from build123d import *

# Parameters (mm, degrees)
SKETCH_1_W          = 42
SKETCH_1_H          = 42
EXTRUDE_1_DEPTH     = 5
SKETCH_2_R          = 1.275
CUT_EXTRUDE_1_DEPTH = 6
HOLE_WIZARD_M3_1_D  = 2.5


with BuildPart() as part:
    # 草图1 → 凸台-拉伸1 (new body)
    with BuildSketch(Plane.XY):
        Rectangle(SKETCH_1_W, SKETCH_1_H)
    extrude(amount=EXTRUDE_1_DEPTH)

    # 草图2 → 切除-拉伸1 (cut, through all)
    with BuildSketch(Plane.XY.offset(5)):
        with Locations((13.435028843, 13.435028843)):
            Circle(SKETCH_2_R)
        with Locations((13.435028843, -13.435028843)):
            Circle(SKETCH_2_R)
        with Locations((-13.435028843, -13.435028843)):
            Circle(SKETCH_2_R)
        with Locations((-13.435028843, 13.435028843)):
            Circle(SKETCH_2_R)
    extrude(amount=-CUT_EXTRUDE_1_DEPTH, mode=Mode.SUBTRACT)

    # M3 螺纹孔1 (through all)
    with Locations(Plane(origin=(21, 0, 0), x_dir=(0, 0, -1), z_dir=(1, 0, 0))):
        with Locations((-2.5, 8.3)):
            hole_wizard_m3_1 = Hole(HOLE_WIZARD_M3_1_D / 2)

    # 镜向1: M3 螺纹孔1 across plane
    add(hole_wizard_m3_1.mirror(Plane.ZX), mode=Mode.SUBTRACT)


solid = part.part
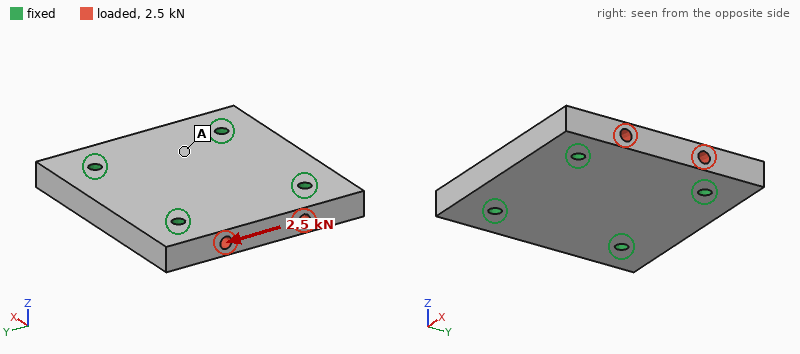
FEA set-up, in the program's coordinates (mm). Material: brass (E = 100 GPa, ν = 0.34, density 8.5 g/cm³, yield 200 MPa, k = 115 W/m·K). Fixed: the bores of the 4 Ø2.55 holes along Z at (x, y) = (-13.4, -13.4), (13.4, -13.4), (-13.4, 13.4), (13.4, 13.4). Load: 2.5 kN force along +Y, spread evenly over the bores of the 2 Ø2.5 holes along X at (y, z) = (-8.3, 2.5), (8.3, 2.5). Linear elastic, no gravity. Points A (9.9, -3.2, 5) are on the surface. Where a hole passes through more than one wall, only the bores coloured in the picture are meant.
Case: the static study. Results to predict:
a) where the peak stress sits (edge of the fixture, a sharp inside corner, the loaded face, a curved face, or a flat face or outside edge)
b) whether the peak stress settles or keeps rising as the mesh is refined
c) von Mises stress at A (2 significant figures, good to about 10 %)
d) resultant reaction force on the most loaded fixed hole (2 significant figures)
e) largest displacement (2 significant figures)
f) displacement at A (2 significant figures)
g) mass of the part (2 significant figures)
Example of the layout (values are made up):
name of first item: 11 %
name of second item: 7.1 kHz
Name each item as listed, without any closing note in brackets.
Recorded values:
where the peak stress sits: edge of the fixture
whether the peak stress settles or keeps rising as the mesh is refined: keeps rising
von Mises stress at A: 3.1 MPa
resultant reaction force on the most loaded fixed hole: 630 N
largest displacement: 1.4 µm
displacement at A: 1.0 µm
mass of the part: 71 g
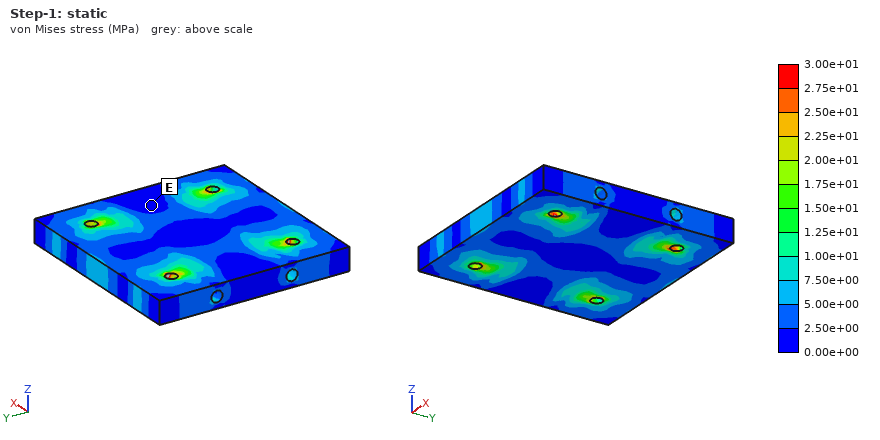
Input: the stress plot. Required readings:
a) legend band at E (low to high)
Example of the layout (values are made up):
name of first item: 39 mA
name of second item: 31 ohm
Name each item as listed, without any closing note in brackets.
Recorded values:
legend band at E: 0.00e+00 to 2.50e+00 MPa
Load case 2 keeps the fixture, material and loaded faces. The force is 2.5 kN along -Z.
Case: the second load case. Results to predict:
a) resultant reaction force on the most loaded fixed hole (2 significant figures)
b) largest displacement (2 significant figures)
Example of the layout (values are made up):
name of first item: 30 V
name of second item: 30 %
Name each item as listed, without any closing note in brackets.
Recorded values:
resultant reaction force on the most loaded fixed hole: 630 N
largest displacement: 8.1 µm
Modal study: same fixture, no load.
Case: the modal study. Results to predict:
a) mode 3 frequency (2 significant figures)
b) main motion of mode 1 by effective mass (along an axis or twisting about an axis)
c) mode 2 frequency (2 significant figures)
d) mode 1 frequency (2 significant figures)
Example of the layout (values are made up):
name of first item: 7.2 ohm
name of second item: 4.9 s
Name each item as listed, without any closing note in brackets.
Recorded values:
mode 3 frequency: 17 kHz
main motion of mode 1 by effective mass: along Z
mode 2 frequency: 17 kHz
mode 1 frequency: 14 kHz
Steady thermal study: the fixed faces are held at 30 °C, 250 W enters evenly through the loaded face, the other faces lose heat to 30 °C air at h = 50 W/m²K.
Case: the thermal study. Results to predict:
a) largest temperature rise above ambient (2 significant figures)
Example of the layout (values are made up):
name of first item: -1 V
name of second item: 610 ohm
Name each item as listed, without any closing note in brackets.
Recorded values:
largest temperature rise above ambient: 60 K
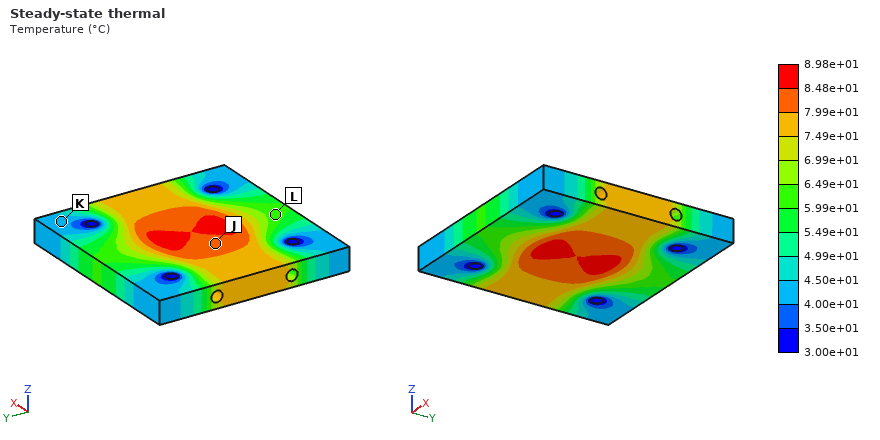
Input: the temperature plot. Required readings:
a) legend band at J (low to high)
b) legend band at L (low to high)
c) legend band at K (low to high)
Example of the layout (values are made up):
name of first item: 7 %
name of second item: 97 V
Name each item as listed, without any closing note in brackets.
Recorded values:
legend band at J: 7.99e+01 to 8.48e+01 °C
legend band at L: 5.99e+01 to 6.49e+01 °C
legend band at K: 4.00e+01 to 4.50e+01 °C
